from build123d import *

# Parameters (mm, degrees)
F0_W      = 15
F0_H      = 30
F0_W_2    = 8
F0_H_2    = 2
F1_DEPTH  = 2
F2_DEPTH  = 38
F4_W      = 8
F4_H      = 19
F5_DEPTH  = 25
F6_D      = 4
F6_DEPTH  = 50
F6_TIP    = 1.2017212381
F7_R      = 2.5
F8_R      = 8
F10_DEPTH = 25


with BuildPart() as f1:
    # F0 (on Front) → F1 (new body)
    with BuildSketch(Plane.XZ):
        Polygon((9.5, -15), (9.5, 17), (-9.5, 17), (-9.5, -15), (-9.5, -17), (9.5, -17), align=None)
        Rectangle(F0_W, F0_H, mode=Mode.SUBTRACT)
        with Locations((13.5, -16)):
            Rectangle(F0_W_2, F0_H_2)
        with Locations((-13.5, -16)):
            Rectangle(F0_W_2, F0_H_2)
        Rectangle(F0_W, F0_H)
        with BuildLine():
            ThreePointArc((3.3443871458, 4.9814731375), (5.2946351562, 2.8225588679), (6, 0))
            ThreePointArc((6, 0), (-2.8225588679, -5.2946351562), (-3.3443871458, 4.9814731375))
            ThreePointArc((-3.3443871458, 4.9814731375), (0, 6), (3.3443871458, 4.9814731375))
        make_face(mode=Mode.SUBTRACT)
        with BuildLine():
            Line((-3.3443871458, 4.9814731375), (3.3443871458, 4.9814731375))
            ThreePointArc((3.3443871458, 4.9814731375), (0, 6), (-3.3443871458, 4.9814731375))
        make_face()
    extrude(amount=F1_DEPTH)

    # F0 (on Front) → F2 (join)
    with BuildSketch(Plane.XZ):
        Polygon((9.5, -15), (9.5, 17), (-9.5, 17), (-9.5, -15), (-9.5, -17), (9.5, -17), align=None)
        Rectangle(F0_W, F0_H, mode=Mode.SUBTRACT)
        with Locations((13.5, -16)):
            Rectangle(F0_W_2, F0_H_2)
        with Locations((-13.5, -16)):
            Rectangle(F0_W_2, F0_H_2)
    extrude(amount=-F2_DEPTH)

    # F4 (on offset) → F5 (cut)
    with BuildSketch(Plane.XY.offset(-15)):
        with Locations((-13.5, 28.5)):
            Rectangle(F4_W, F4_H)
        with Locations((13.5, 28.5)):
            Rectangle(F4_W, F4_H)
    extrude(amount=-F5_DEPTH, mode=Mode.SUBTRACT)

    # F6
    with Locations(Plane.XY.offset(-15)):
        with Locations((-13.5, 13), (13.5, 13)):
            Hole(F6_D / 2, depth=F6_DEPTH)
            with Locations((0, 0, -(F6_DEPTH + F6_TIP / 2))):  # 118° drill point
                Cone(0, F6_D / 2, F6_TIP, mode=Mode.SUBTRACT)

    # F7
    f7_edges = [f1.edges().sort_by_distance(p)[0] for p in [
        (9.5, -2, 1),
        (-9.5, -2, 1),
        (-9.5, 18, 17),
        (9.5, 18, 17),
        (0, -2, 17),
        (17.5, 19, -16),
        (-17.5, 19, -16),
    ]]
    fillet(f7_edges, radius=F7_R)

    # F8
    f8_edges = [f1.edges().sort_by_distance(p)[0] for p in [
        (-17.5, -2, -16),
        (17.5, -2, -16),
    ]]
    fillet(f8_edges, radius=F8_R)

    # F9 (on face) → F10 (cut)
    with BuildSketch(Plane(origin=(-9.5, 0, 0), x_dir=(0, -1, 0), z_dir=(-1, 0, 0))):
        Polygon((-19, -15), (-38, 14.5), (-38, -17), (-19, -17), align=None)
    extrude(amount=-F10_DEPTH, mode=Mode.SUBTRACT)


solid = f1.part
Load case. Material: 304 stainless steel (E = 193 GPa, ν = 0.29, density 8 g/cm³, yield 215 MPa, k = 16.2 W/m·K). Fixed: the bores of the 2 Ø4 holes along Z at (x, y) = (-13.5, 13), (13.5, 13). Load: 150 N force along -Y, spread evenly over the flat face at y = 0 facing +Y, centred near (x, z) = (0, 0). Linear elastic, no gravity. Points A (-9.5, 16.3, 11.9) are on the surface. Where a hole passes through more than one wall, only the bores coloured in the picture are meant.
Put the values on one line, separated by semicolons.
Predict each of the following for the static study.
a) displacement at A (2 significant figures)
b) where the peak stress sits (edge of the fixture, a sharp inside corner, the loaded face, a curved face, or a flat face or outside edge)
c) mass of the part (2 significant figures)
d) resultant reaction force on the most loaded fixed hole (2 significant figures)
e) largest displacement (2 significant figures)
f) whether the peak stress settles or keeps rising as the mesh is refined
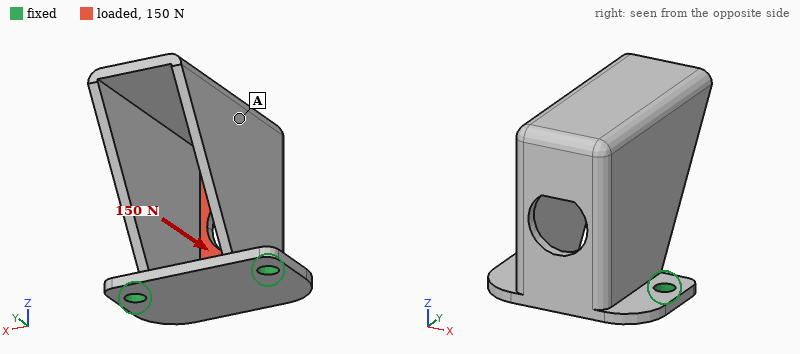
29 µm; edge of the fixture; 56 g; 77 N; 43 µm; keeps rising
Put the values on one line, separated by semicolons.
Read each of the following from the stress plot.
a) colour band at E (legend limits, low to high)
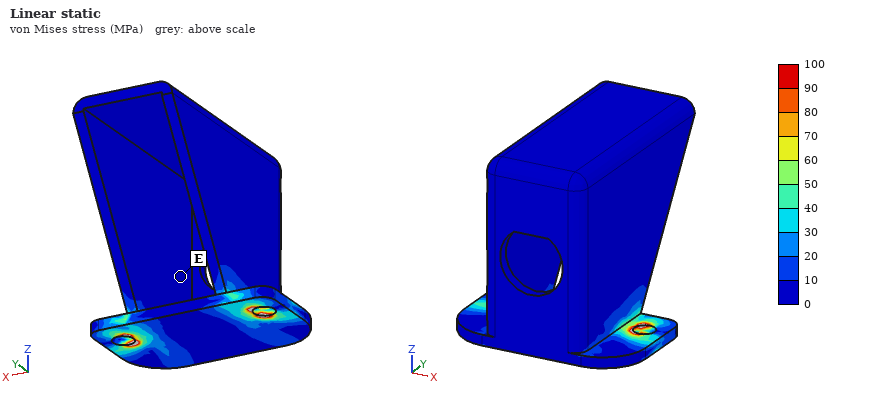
0 to 10 MPa
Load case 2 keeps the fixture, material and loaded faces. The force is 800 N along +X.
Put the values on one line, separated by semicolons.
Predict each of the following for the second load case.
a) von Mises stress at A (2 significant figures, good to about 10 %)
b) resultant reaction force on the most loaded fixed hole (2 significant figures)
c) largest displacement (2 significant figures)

28 MPa; 790 N; 97 µm
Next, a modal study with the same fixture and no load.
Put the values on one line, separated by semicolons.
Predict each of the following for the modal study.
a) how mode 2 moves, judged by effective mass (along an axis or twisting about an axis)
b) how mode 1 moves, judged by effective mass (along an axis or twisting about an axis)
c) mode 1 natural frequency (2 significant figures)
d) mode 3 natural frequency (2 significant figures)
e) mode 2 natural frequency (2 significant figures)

along X; along Y; 1400 Hz; 6600 Hz; 1600 Hz
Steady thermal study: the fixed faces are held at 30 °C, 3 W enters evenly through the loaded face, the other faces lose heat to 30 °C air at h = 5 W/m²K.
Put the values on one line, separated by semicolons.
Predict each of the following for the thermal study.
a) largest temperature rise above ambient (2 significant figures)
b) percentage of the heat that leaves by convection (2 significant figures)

41 K; 26 %
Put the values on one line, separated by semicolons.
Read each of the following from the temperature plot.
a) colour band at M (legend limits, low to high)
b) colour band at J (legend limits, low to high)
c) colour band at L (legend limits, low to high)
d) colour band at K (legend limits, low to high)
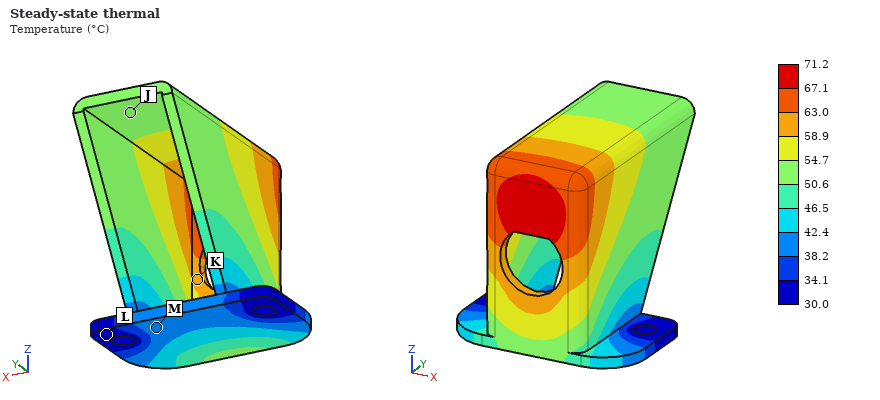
38.2 to 42.4 °C; 50.6 to 54.7 °C; 30.0 to 34.1 °C; 58.9 to 63.0 °C
